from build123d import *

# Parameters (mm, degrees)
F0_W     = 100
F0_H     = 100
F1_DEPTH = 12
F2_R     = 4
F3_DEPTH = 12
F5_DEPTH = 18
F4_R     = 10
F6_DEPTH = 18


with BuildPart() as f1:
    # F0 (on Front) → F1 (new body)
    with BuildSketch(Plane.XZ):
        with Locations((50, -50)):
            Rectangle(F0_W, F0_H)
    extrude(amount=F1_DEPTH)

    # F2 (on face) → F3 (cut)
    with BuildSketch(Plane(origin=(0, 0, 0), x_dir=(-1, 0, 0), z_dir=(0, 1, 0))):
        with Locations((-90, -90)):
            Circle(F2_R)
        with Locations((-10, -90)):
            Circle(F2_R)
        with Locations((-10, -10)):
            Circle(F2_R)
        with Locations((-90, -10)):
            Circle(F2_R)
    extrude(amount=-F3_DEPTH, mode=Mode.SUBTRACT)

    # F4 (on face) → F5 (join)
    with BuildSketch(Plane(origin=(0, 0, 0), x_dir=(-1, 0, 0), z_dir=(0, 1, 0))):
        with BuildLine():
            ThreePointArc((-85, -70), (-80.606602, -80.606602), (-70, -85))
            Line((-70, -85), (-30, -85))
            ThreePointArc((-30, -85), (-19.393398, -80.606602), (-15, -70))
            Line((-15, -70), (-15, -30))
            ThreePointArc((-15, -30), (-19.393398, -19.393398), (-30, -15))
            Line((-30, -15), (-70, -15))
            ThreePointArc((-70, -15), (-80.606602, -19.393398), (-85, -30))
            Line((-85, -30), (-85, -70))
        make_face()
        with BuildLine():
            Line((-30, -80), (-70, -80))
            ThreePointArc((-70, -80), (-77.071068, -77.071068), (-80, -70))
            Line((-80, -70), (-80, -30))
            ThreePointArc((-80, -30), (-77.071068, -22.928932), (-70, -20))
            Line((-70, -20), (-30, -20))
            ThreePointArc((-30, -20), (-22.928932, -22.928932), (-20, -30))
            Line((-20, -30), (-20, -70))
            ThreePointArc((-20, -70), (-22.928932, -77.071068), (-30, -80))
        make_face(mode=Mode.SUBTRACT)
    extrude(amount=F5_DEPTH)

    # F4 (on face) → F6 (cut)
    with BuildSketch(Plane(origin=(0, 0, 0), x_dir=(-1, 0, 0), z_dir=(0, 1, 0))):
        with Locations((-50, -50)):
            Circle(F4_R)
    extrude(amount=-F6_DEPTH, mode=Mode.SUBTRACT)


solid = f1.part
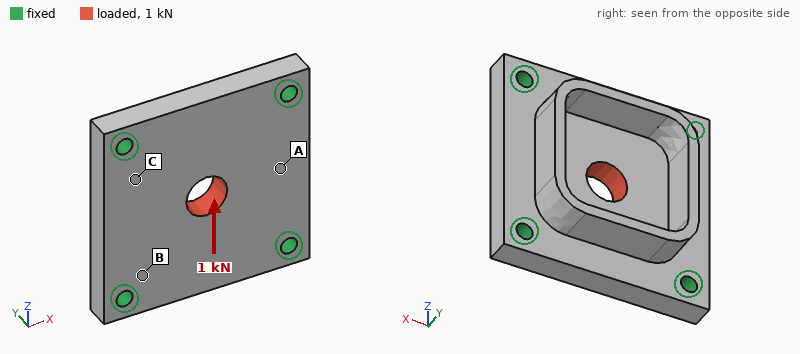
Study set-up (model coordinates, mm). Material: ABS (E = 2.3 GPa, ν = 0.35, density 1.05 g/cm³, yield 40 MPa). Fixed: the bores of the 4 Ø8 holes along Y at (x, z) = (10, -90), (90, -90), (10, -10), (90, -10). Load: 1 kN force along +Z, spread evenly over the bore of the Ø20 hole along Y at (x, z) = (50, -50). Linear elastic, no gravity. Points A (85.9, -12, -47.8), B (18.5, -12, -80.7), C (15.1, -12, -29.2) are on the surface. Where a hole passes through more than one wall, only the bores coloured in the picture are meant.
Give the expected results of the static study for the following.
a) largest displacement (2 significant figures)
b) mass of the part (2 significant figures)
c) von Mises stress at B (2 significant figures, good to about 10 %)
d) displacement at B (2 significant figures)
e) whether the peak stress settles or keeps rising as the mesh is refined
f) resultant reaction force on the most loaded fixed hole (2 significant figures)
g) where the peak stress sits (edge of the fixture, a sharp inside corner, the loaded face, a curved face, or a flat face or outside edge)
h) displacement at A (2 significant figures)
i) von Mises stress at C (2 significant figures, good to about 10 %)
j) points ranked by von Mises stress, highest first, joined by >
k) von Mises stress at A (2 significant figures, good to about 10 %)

27 µm
140 g
1.1 MPa
6.3 µm
keeps rising
280 N
edge of the fixture
7.9 µm
0.72 MPa
B > C > A
0.34 MPa
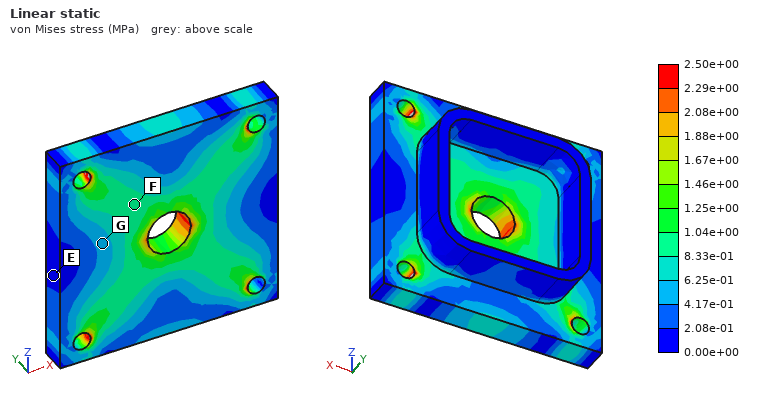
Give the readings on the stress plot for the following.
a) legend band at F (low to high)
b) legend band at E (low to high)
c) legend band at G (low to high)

8.33e-01 to 1.04e+00 MPa
0.00e+00 to 2.08e-01 MPa
4.17e-01 to 6.25e-01 MPa
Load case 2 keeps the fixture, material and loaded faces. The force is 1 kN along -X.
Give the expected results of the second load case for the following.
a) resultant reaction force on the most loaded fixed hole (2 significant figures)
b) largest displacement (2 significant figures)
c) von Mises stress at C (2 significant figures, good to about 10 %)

280 N
27 µm
0.75 MPa
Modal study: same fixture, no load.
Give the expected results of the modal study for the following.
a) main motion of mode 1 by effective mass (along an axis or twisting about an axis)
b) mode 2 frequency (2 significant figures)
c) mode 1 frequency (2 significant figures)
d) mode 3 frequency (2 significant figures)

along Y
2900 Hz
2000 Hz
2900 Hz
